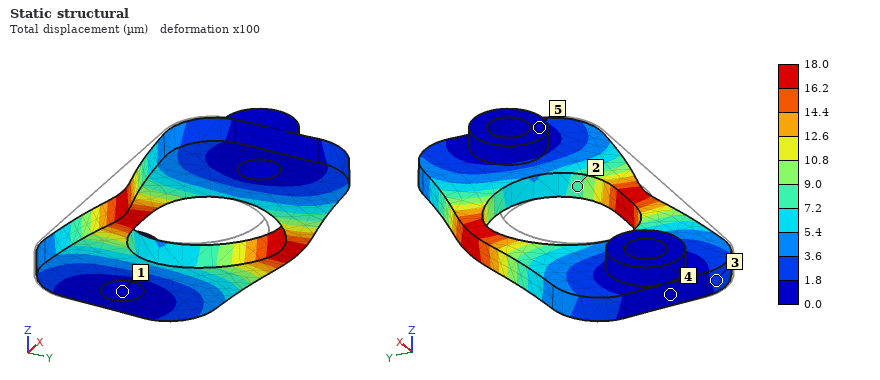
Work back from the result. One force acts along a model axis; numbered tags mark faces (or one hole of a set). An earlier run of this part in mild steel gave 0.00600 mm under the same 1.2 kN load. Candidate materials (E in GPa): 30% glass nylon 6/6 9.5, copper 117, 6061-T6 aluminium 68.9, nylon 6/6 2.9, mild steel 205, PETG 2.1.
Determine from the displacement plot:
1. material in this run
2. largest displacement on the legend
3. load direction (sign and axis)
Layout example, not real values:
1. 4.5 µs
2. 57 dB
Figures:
1. 6061-T6 aluminium
2. 18.0 µm
3. +Y
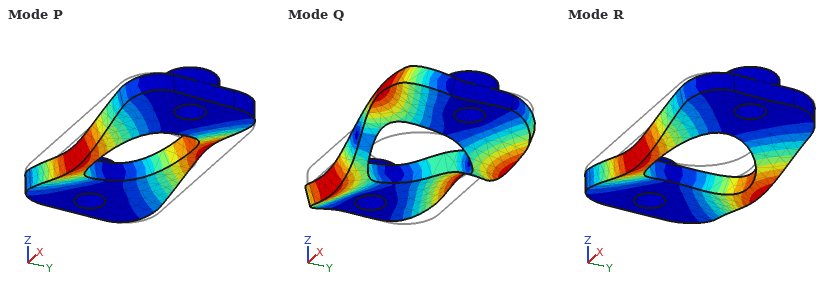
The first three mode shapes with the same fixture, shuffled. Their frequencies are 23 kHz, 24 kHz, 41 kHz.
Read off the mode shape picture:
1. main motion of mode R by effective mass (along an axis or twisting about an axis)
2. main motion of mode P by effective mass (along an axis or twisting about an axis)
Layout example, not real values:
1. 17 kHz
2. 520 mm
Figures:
1. along Z
2. twisting about X
